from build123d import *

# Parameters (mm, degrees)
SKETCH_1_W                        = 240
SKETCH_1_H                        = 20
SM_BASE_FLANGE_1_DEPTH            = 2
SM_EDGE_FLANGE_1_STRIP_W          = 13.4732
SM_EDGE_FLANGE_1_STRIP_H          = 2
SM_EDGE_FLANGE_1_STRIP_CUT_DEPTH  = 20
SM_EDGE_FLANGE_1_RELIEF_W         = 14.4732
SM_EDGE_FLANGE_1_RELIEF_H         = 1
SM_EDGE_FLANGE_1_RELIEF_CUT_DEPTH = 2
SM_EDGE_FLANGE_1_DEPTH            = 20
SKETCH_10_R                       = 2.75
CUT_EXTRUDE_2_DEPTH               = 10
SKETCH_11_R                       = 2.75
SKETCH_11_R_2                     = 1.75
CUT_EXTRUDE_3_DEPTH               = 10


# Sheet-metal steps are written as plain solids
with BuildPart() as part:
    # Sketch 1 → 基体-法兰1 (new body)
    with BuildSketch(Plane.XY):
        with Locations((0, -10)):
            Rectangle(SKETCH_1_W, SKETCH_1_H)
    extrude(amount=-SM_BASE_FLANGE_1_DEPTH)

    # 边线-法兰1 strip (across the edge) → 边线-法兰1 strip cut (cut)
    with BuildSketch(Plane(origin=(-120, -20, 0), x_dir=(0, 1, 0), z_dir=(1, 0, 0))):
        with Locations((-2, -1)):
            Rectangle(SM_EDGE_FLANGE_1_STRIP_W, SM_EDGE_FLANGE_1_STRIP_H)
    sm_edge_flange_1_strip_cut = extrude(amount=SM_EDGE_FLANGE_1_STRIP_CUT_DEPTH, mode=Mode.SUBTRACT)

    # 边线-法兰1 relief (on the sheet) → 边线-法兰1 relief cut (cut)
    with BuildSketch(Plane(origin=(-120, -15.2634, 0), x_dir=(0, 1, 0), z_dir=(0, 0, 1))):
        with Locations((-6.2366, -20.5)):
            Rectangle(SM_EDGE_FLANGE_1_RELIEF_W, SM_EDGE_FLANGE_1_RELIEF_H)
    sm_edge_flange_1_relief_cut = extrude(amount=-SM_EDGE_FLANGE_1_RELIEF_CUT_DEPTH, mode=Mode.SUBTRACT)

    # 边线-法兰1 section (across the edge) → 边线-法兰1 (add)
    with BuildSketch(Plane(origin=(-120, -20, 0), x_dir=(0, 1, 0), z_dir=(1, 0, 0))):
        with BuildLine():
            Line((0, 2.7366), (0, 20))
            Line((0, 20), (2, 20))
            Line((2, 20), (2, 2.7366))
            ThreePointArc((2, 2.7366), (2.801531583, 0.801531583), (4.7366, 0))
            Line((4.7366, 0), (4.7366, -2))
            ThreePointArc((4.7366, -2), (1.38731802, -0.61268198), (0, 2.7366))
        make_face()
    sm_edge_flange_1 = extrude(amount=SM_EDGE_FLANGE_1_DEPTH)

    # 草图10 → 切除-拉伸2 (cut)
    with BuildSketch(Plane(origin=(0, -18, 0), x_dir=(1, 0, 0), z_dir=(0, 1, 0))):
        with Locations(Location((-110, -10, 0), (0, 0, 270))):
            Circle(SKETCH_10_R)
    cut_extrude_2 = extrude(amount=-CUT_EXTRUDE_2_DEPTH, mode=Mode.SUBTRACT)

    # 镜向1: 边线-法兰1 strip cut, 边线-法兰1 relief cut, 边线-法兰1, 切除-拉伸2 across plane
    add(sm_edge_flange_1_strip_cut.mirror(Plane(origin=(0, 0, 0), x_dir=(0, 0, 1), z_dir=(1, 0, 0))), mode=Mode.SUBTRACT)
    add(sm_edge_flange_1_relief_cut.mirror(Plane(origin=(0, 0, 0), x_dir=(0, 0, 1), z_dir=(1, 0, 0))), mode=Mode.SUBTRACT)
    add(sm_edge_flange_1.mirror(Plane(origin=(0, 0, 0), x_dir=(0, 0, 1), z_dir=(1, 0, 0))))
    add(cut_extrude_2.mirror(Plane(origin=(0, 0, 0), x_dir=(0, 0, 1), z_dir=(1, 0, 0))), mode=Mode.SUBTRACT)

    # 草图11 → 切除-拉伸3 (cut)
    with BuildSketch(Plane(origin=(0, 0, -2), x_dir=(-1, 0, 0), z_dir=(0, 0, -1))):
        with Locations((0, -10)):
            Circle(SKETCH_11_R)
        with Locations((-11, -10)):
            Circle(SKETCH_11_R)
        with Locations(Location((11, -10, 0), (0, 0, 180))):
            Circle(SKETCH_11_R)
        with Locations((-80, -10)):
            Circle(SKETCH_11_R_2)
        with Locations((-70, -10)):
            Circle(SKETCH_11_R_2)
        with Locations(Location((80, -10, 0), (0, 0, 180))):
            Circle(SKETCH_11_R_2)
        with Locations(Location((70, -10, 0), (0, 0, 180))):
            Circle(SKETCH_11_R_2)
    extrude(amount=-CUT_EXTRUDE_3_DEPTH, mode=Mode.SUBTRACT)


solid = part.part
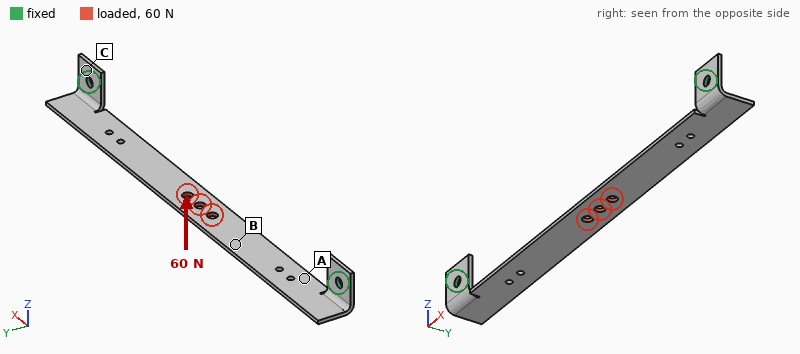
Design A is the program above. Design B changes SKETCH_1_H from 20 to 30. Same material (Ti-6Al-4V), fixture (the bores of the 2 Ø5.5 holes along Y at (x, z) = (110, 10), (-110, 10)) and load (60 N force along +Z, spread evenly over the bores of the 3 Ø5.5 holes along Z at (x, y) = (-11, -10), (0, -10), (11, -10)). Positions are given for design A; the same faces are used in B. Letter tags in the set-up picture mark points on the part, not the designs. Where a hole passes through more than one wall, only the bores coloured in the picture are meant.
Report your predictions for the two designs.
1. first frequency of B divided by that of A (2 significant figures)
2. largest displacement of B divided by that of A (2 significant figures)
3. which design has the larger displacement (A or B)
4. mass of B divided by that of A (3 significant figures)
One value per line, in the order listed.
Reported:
0.94
0.72
A
1.41
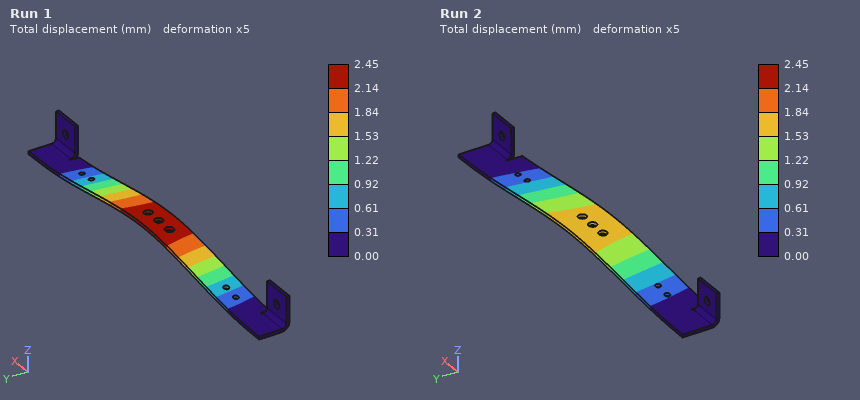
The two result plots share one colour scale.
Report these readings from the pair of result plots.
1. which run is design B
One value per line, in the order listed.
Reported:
Run 2
